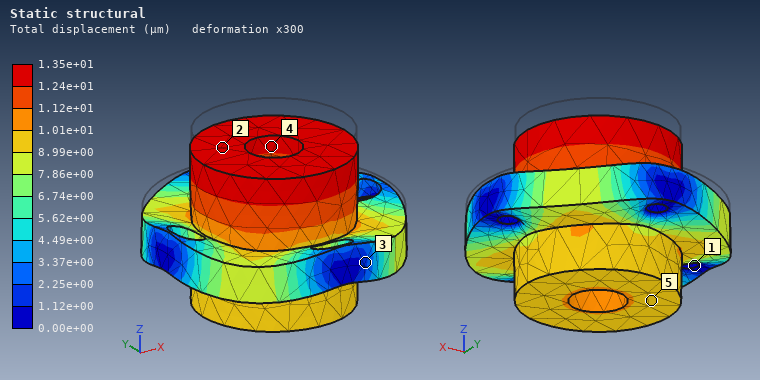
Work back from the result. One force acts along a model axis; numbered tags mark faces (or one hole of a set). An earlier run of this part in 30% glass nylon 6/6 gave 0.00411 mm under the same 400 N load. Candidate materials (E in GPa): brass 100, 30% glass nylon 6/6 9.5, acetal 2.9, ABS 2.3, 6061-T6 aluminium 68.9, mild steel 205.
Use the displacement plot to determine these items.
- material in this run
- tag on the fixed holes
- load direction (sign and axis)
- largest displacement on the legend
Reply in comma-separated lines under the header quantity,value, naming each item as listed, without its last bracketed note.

quantity,value
material in this run,acetal
tag on the fixed holes,1
load direction,-Z
largest displacement on the legend,1.35e+01 µm
